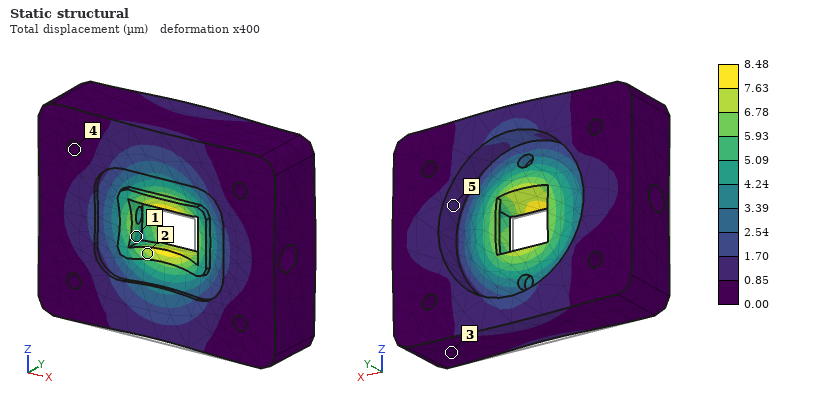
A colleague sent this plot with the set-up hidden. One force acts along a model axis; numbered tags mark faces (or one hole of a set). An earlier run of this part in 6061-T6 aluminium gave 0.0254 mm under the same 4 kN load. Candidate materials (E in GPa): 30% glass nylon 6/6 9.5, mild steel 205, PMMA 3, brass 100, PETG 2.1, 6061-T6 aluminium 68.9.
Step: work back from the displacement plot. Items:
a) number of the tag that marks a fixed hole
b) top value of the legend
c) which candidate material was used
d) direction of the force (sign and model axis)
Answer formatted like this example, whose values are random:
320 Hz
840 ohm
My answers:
4
8.48 µm
mild steel
+Y
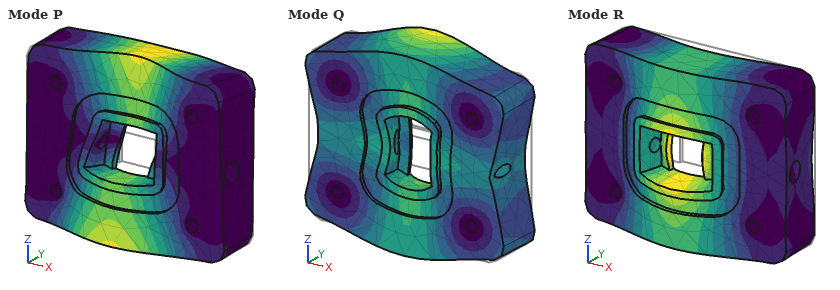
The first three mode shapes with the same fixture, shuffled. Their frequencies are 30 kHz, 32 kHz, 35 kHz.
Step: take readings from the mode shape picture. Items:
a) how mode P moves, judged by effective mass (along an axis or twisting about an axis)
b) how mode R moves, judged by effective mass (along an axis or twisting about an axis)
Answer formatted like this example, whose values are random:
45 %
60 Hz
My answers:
twisting about X
along Y
